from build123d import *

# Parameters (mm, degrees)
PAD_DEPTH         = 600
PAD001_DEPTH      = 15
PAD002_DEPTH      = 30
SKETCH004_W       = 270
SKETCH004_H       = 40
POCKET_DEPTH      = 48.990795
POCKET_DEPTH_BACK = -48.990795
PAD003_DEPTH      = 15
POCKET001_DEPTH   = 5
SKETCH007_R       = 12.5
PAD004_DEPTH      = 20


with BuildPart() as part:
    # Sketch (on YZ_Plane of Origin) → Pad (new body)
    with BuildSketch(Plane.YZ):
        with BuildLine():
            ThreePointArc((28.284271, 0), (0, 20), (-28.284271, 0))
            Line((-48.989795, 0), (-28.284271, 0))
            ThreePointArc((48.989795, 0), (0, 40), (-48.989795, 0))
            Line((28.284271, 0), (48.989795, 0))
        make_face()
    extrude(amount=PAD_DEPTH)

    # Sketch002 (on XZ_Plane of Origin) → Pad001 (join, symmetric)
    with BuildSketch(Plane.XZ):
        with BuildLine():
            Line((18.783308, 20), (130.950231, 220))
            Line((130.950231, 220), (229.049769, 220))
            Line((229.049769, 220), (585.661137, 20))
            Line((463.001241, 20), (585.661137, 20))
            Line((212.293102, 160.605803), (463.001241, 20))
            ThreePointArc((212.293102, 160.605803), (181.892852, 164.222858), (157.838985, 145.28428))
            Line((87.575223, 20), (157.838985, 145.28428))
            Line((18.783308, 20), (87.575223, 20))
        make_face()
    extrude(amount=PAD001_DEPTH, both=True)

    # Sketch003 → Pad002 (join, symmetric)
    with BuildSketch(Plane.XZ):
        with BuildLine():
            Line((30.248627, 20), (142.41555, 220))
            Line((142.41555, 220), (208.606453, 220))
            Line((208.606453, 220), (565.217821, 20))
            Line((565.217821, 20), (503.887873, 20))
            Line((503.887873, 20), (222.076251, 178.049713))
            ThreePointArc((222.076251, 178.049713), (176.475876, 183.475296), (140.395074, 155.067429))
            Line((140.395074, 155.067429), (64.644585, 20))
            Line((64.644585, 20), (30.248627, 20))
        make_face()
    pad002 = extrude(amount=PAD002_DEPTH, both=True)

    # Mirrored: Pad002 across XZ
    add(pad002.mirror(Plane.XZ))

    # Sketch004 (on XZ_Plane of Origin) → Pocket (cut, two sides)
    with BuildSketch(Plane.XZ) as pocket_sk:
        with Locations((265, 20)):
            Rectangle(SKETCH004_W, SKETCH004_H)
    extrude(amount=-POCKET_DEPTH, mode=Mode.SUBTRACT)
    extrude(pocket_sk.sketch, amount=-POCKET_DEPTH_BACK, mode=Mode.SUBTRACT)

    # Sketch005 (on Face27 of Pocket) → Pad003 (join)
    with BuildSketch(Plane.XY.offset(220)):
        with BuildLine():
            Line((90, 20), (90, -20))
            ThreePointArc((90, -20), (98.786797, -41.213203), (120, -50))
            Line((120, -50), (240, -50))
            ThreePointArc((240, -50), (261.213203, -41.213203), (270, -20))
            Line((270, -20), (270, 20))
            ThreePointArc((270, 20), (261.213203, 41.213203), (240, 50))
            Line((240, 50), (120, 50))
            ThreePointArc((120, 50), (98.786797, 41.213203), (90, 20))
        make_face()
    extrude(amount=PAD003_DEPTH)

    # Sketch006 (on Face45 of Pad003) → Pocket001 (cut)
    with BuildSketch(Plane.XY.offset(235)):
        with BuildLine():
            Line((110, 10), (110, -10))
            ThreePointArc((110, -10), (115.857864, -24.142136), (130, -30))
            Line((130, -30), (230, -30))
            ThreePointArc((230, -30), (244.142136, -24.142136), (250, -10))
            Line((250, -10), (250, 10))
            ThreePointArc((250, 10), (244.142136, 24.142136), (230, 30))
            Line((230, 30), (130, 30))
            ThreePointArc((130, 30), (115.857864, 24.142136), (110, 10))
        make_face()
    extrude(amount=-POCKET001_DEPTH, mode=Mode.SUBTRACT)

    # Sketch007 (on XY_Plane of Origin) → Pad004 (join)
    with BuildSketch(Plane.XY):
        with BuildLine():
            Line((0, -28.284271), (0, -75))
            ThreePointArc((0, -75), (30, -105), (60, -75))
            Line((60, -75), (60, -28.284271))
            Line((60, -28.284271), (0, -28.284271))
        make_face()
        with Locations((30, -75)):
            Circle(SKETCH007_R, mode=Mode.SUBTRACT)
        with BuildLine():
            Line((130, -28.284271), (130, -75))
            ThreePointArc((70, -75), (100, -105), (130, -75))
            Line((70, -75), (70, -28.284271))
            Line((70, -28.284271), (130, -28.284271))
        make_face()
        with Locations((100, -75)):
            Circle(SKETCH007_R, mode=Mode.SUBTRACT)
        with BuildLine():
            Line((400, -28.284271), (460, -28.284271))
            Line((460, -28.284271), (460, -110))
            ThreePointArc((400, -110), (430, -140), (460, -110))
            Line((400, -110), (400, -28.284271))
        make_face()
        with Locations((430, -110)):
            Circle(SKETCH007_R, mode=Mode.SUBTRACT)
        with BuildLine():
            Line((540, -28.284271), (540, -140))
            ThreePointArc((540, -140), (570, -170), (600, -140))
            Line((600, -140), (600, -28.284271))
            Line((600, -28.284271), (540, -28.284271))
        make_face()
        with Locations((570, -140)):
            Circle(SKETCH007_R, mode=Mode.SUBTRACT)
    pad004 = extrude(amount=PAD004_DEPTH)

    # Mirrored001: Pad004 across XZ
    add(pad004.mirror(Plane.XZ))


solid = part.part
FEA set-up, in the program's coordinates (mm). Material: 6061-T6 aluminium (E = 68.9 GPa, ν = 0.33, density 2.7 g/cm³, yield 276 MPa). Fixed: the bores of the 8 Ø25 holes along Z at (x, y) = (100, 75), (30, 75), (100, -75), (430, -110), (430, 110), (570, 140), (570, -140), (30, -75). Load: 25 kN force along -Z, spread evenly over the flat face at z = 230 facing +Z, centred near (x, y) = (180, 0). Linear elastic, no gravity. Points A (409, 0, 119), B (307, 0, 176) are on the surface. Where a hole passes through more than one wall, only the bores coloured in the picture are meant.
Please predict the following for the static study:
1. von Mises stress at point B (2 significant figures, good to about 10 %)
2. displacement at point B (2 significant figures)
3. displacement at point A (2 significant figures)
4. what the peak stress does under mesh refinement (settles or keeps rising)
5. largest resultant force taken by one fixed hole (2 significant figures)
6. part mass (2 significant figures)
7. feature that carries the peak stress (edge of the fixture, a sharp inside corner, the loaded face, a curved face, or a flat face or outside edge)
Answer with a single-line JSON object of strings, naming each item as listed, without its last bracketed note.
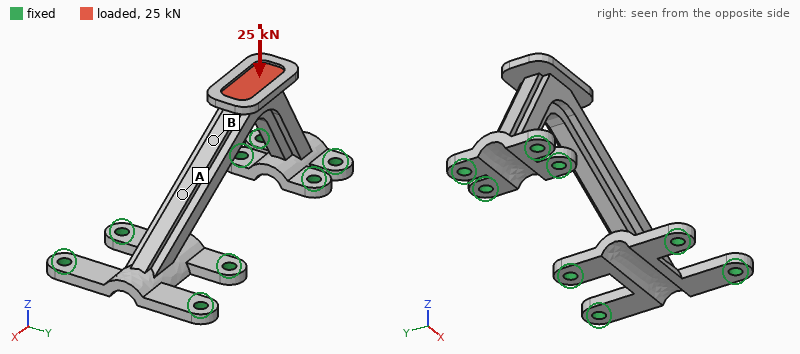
{"von Mises stress at point B": "9.3 MPa", "displacement at point B": "0.082 mm", "displacement at point A": "0.057 mm", "what the peak stress does under mesh refinement": "keeps rising", "largest resultant force taken by one fixed hole": "8.8 kN", "part mass": "8.4 kg", "feature that carries the peak stress": "edge of the fixture"}
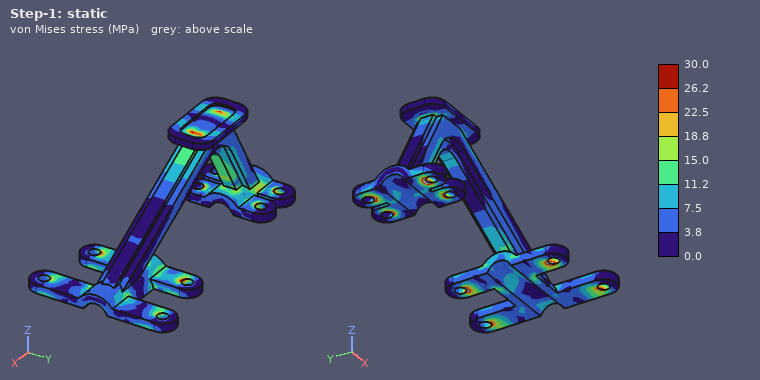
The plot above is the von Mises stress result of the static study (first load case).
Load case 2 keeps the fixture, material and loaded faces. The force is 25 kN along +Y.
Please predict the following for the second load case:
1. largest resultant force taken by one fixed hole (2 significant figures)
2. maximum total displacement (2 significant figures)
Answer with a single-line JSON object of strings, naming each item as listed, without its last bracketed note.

{"largest resultant force taken by one fixed hole": "21 kN", "maximum total displacement": "2.4 mm"}
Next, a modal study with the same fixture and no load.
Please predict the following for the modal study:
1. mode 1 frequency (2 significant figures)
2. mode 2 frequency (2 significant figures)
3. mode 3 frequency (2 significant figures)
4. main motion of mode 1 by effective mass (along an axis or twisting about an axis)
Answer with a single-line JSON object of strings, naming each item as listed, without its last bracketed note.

{"mode 1 frequency": "420 Hz", "mode 2 frequency": "980 Hz", "mode 3 frequency": "1200 Hz", "main motion of mode 1 by effective mass": "along Y"}
